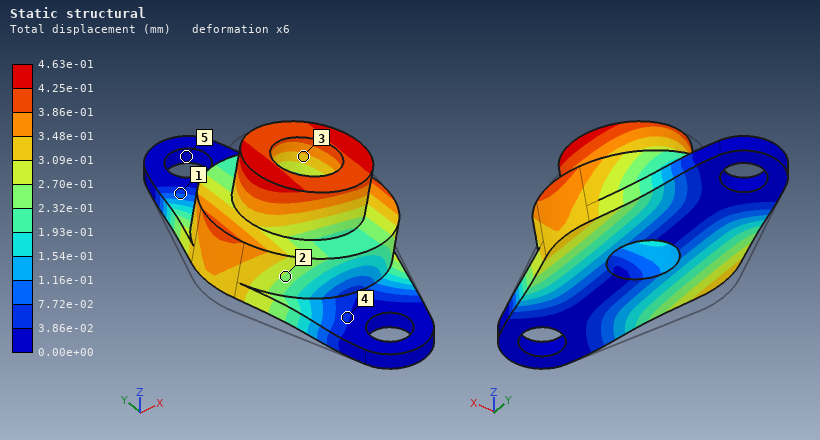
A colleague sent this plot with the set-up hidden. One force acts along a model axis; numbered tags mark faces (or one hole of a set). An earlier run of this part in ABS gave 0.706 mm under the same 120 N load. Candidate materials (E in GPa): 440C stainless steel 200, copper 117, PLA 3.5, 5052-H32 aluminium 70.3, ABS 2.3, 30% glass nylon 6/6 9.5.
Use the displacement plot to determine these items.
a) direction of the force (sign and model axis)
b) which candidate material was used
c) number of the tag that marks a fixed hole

+X
PLA
5
